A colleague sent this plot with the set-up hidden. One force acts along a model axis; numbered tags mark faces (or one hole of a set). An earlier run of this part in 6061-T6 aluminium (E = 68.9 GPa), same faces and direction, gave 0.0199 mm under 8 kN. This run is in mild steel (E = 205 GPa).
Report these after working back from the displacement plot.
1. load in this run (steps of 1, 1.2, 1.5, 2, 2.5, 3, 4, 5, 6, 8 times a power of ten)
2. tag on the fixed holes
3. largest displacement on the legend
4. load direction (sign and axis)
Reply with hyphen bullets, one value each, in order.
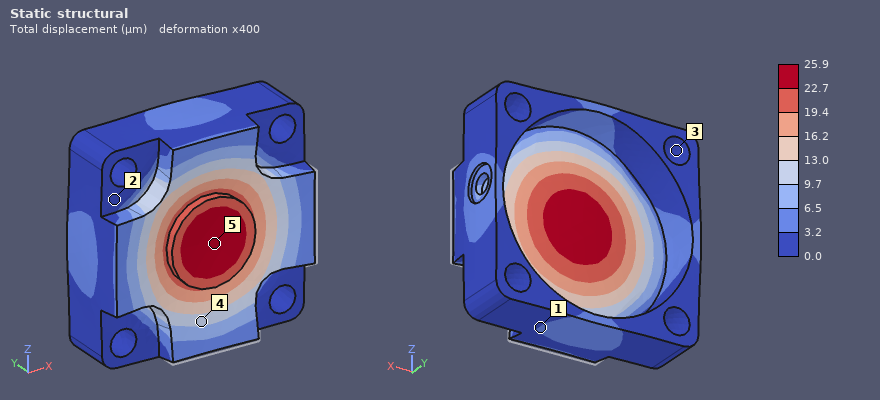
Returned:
- 30 kN
- 3
- 25.9 µm
- +Y
